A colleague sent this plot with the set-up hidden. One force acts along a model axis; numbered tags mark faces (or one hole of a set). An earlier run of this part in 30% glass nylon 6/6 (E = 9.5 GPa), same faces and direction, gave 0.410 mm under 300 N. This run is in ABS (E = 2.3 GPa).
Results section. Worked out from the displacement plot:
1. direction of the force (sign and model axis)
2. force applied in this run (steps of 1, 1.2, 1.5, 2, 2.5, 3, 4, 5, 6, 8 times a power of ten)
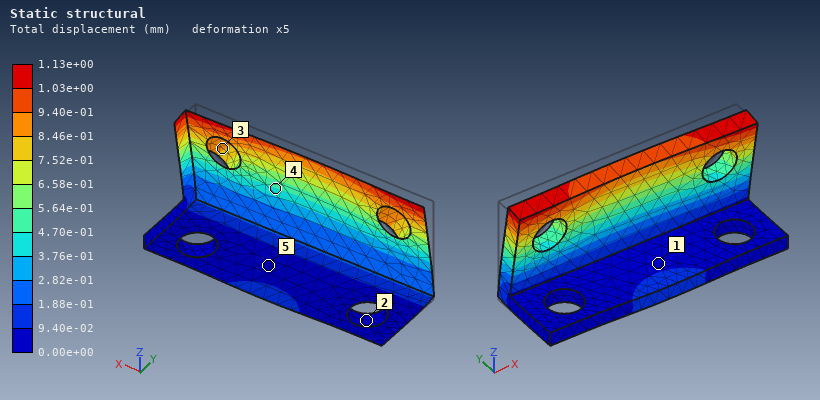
-Y
200 N
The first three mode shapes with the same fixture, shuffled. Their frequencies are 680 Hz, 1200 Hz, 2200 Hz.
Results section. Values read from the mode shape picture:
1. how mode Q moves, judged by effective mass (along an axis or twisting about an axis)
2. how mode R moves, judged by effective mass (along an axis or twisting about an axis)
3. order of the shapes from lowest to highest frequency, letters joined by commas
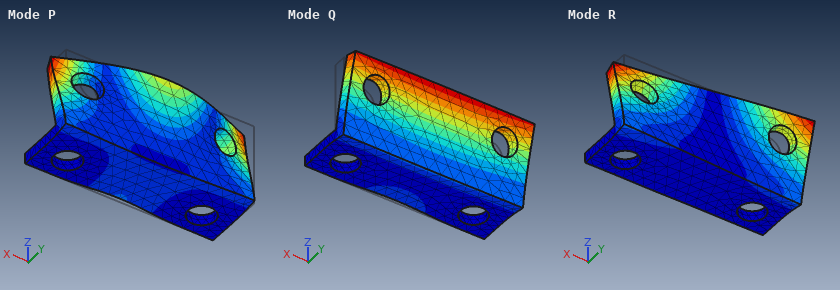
along Y
twisting about Z
Q, R, P
